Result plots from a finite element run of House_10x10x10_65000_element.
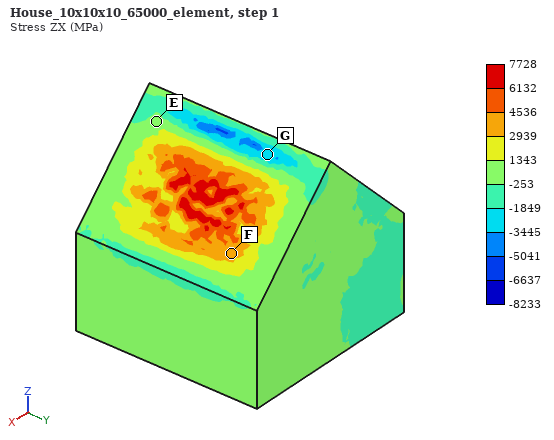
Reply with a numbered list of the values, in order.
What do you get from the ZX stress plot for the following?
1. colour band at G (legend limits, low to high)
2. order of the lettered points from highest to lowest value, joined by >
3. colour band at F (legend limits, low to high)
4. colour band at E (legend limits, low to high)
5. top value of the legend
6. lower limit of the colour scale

1. -3445 to -1849 MPa
2. F > E > G
3. 2939 to 4536 MPa
4. -253 to 1343 MPa
5. 7728 MPa
6. -8233 MPa
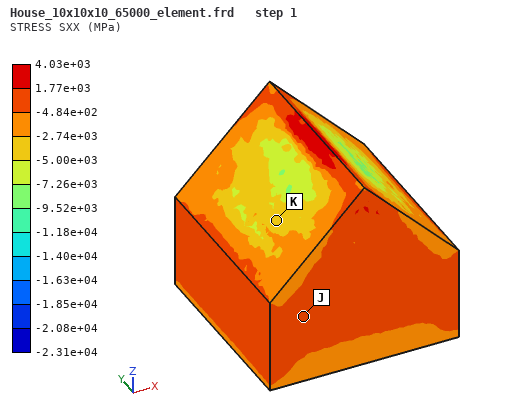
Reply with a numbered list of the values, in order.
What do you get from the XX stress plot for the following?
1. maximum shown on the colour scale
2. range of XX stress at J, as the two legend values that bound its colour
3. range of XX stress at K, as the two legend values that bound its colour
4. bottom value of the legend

1. 4.03e+03 MPa
2. -4.84e+02 to 1.77e+03 MPa
3. -5.00e+03 to -2.74e+03 MPa
4. -2.31e+04 MPa
